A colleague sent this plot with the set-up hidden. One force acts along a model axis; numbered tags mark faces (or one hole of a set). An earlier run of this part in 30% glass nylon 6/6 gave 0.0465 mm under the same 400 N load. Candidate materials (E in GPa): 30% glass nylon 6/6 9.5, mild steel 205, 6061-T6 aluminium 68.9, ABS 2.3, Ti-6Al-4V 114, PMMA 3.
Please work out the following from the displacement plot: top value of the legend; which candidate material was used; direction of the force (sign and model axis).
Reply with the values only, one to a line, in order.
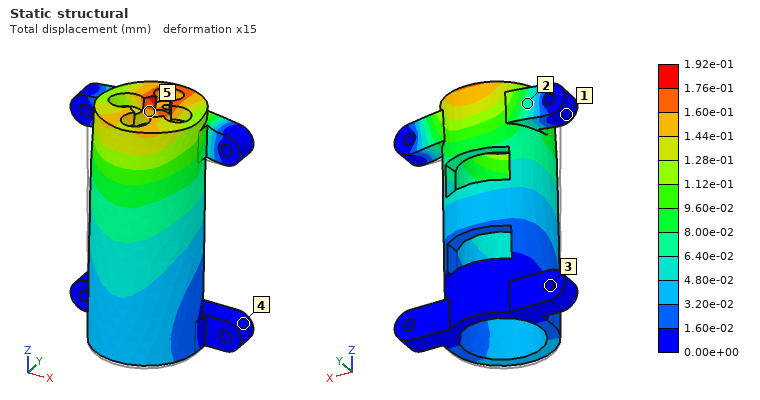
1.92e-01 mm
ABS
+Y
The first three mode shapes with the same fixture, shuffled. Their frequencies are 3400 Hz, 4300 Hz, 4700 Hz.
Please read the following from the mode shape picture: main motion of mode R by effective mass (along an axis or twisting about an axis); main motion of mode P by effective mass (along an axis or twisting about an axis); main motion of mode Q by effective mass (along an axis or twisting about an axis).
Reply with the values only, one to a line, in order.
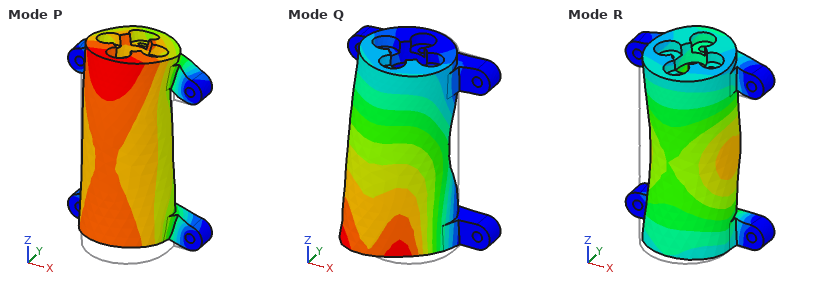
along Y
along Z
along X
